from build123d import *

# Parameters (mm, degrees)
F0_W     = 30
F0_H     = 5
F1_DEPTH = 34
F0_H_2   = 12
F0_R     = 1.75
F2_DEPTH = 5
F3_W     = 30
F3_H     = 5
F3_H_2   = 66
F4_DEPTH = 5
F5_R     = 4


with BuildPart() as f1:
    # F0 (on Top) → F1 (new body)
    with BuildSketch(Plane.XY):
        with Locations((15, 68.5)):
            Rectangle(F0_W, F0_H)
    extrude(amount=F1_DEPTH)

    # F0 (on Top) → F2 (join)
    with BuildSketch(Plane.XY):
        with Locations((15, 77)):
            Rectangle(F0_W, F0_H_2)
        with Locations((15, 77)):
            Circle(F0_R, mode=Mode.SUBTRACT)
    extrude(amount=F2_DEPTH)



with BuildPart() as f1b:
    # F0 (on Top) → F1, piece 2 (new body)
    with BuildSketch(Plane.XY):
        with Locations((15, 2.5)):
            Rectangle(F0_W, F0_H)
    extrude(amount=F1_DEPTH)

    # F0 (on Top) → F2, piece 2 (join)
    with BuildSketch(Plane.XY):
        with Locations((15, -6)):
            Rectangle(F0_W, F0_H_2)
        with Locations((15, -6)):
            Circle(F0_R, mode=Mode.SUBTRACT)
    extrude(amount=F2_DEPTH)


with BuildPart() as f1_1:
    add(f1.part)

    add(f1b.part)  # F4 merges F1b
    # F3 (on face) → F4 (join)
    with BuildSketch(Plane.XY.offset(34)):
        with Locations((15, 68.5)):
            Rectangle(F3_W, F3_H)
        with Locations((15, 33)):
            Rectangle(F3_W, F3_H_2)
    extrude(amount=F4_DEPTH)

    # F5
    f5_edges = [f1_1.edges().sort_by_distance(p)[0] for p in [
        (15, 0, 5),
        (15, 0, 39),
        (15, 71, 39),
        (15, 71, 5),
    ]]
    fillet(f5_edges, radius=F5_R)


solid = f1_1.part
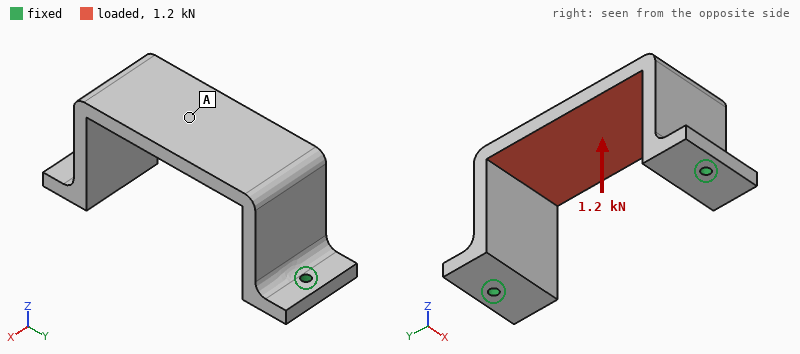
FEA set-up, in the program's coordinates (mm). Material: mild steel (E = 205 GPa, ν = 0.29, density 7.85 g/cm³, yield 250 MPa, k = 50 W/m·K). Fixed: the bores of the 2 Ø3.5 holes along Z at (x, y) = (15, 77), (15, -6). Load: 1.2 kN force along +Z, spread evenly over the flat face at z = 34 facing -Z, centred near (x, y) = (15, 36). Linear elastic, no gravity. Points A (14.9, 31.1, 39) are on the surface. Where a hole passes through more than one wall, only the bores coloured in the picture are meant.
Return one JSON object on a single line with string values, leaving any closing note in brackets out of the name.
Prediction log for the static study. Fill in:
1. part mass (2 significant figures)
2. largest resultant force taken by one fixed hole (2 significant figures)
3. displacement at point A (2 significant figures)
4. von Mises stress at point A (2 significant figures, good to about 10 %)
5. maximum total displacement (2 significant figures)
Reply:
{"part mass": "190 g", "largest resultant force taken by one fixed hole": "670 N", "displacement at point A": "25 µm", "von Mises stress at point A": "35 MPa", "maximum total displacement": "27 µm"}
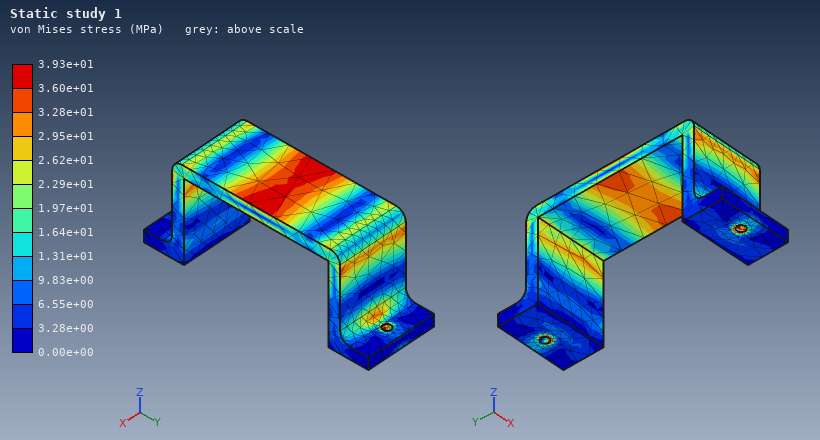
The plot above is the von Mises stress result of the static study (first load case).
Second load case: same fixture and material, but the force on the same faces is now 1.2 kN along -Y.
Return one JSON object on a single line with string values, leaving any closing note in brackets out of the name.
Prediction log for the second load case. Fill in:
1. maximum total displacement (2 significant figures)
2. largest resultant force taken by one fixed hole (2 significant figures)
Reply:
{"maximum total displacement": "69 µm", "largest resultant force taken by one fixed hole": "650 N"}
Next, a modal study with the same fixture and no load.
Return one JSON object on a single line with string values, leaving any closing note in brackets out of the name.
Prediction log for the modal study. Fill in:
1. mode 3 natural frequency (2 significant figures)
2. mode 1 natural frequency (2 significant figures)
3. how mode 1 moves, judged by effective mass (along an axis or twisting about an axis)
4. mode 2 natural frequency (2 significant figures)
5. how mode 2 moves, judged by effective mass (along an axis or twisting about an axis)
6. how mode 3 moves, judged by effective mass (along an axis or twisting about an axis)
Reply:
{"mode 3 natural frequency": "3100 Hz", "mode 1 natural frequency": "1800 Hz", "how mode 1 moves, judged by effective mass": "along X", "mode 2 natural frequency": "2100 Hz", "how mode 2 moves, judged by effective mass": "along Y", "how mode 3 moves, judged by effective mass": "twisting about Z"}
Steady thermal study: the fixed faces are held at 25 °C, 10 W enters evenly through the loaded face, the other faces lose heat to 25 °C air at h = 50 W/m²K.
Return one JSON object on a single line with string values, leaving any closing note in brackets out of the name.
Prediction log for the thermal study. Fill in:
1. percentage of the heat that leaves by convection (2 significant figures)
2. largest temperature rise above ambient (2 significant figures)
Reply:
{"percentage of the heat that leaves by convection": "52 %", "largest temperature rise above ambient": "24 K"}
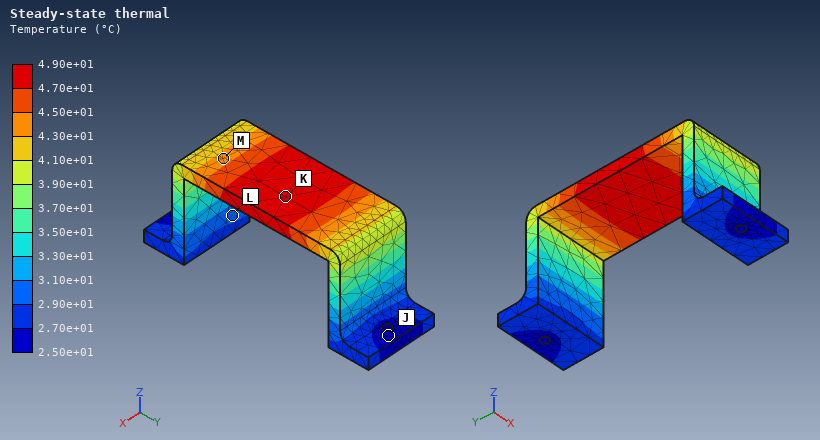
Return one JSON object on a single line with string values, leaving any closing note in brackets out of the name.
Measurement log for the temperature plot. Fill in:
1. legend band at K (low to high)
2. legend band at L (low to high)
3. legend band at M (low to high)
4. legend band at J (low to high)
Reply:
{"legend band at K": "4.70e+01 to 4.90e+01 °C", "legend band at L": "2.90e+01 to 3.10e+01 °C", "legend band at M": "4.30e+01 to 4.50e+01 °C", "legend band at J": "2.50e+01 to 2.70e+01 °C"}
